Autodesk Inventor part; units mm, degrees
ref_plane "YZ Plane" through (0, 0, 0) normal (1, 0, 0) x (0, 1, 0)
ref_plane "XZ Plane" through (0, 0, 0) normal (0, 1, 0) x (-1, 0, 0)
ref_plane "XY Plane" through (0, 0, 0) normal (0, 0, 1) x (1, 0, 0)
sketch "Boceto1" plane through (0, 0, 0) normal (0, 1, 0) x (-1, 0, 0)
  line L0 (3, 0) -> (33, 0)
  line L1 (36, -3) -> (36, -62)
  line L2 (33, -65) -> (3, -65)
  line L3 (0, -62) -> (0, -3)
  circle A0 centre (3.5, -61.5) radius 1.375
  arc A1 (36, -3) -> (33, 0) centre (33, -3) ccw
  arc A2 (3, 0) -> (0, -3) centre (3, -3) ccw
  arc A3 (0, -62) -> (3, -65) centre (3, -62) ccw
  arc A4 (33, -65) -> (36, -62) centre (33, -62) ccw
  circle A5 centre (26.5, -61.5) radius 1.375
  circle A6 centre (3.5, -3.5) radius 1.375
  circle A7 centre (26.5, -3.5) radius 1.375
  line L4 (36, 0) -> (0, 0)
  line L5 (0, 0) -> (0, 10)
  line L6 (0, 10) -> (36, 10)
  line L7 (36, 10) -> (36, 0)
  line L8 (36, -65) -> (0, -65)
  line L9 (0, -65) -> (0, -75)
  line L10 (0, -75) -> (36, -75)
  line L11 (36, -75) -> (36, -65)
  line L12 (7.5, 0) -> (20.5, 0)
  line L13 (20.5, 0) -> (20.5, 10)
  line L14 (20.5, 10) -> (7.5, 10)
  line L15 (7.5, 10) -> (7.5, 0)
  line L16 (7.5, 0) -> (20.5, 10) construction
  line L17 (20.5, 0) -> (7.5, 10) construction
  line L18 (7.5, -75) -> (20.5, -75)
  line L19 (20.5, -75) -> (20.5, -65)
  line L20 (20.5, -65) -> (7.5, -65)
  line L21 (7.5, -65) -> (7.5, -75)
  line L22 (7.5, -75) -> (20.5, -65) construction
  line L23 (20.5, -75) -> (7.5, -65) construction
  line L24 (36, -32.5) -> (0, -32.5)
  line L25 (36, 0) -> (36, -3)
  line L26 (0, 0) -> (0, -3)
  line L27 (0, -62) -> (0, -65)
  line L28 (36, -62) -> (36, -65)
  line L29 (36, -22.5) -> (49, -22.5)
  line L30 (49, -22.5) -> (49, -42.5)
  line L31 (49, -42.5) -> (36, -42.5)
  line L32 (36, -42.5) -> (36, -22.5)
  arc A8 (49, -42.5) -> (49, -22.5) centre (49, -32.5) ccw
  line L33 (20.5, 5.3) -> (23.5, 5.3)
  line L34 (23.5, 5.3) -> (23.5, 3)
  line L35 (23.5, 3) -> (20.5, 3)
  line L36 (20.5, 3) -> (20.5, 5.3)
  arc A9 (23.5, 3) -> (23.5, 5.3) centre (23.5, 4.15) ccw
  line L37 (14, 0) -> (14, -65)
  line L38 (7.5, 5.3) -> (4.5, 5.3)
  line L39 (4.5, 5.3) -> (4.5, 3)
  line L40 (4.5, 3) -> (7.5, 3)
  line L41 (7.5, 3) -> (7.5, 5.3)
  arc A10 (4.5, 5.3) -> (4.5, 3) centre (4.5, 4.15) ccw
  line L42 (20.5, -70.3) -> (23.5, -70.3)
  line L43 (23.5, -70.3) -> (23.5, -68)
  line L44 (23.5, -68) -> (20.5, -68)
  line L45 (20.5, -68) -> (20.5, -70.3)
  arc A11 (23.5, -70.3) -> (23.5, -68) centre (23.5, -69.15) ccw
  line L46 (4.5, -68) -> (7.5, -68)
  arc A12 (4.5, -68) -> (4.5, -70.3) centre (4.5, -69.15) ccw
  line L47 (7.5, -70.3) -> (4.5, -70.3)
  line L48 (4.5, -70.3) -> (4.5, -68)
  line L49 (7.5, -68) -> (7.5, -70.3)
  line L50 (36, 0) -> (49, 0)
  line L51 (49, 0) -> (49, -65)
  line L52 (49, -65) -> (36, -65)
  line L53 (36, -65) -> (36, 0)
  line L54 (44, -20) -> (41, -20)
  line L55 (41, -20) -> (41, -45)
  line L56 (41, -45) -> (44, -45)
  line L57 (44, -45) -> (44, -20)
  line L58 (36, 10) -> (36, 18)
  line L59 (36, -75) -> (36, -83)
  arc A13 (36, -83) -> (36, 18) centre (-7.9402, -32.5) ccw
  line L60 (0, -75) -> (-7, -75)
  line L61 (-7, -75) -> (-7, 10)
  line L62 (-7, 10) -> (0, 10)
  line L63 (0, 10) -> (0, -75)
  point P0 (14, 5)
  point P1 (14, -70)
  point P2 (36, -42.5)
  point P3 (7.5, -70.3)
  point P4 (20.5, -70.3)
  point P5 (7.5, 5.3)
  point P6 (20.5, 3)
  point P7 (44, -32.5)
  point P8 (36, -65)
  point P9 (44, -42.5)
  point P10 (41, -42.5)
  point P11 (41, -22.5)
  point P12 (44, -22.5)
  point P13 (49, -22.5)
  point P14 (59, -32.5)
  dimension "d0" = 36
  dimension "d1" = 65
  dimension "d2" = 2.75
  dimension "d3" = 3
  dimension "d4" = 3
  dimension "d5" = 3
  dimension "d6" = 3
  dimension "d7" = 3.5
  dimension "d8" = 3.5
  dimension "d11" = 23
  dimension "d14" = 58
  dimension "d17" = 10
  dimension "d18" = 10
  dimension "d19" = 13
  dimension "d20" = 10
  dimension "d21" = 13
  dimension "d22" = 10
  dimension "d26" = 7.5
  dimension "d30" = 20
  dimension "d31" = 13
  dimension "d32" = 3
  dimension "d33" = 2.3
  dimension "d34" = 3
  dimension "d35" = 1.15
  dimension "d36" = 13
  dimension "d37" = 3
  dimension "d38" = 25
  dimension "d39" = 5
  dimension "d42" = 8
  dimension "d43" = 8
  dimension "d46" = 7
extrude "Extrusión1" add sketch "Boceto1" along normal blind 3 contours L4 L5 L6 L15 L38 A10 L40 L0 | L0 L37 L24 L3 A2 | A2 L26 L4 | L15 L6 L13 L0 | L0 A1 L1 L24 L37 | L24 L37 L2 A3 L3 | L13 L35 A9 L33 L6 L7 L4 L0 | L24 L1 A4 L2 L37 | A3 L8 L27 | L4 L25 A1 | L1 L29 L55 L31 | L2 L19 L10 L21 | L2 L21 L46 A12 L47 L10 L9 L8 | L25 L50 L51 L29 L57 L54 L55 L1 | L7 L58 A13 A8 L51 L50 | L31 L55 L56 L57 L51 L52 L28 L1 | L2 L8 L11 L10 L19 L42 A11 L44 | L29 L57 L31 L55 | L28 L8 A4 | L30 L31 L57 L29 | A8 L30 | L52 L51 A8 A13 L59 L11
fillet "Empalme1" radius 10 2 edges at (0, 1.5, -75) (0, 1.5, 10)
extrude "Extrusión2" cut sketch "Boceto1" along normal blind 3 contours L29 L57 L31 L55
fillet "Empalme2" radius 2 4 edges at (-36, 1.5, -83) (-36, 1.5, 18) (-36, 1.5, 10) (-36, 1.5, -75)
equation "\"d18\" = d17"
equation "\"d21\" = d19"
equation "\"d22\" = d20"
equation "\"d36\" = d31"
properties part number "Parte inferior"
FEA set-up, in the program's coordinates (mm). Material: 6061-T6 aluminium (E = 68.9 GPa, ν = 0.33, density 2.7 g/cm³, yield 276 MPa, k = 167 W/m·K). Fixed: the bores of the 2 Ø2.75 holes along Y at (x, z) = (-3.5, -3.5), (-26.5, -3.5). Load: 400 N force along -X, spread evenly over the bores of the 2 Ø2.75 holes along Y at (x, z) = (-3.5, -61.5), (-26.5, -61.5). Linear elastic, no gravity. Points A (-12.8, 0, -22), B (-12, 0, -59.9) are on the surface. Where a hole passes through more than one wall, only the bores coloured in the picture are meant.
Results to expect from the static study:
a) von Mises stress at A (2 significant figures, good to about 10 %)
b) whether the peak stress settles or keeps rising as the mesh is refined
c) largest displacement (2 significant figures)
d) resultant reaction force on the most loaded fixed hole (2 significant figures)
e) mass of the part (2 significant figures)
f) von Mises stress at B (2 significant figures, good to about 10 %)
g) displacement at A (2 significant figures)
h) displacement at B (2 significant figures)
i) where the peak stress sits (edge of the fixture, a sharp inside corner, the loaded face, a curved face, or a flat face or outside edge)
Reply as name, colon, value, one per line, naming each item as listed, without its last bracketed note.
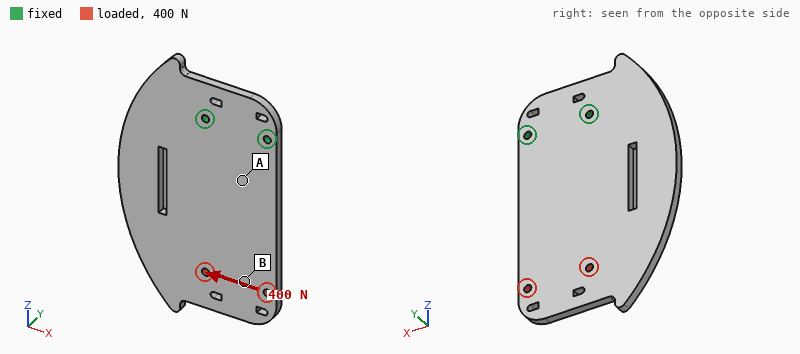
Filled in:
von Mises stress at A: 12 MPa
whether the peak stress settles or keeps rising as the mesh is refined: keeps rising
largest displacement: 52 µm
resultant reaction force on the most loaded fixed hole: 980 N
mass of the part: 36 g
von Mises stress at B: 4.8 MPa
displacement at A: 10.0 µm
displacement at B: 38 µm
where the peak stress sits: edge of the fixture
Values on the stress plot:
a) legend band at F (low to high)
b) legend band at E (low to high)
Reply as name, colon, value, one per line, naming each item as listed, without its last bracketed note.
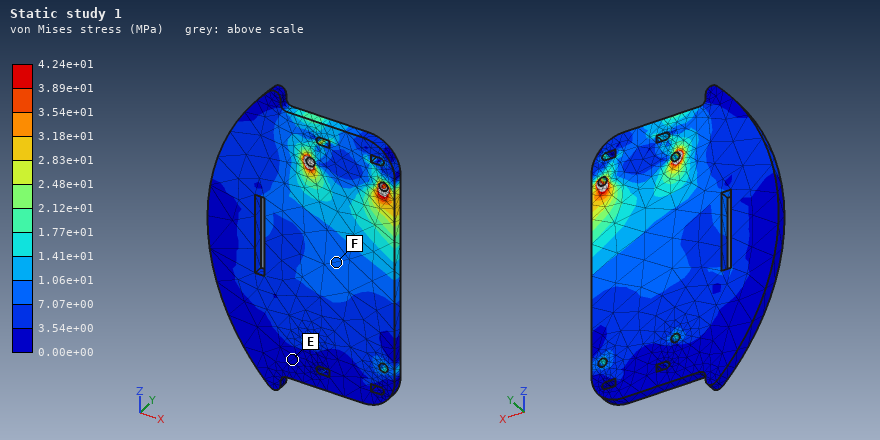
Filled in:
legend band at F: 7.07e+00 to 1.06e+01 MPa
legend band at E: 0.00e+00 to 3.54e+00 MPa
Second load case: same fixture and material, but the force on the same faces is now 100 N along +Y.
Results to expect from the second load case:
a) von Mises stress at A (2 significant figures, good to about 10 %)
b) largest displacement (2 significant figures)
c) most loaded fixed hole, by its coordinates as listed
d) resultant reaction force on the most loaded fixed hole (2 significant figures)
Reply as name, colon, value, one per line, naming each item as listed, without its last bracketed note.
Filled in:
von Mises stress at A: 52 MPa
largest displacement: 1.3 mm
most loaded fixed hole, by its coordinates as listed: (-26.5, -3.5)
resultant reaction force on the most loaded fixed hole: 55 N
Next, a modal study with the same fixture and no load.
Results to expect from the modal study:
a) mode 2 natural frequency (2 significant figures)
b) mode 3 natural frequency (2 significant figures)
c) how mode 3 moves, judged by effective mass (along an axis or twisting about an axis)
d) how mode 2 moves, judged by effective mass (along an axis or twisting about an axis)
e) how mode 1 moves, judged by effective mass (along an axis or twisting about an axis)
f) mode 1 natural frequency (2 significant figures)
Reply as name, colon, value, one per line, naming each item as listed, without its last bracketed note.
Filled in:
mode 2 natural frequency: 1200 Hz
mode 3 natural frequency: 2500 Hz
how mode 3 moves, judged by effective mass: along Y
how mode 2 moves, judged by effective mass: twisting about Z
how mode 1 moves, judged by effective mass: along Y
mode 1 natural frequency: 450 Hz
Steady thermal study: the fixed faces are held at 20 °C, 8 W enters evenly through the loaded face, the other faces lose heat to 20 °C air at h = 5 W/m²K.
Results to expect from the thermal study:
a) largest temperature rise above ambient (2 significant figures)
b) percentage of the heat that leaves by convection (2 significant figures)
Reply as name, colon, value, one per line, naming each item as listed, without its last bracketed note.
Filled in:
largest temperature rise above ambient: 23 K
percentage of the heat that leaves by convection: 6.5 %
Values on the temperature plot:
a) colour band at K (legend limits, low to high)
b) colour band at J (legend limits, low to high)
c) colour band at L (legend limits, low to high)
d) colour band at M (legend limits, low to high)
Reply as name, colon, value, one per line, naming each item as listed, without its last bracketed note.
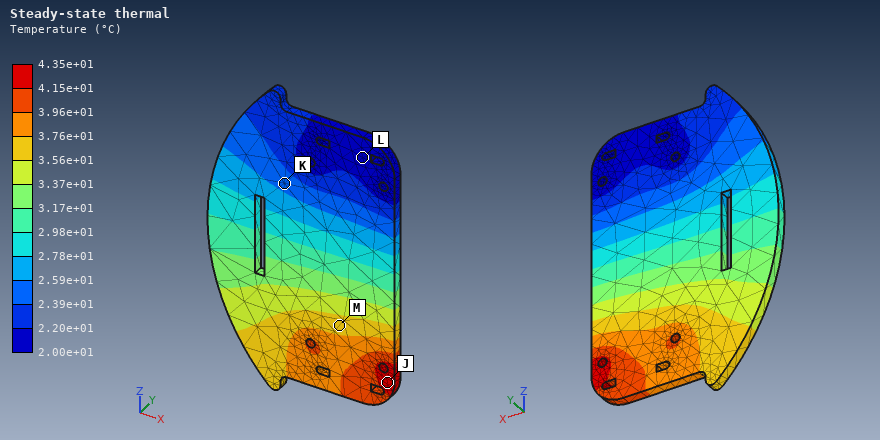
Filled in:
colour band at K: 2.39e+01 to 2.59e+01 °C
colour band at J: 4.15e+01 to 4.35e+01 °C
colour band at L: 2.00e+01 to 2.20e+01 °C
colour band at M: 3.56e+01 to 3.76e+01 °C
